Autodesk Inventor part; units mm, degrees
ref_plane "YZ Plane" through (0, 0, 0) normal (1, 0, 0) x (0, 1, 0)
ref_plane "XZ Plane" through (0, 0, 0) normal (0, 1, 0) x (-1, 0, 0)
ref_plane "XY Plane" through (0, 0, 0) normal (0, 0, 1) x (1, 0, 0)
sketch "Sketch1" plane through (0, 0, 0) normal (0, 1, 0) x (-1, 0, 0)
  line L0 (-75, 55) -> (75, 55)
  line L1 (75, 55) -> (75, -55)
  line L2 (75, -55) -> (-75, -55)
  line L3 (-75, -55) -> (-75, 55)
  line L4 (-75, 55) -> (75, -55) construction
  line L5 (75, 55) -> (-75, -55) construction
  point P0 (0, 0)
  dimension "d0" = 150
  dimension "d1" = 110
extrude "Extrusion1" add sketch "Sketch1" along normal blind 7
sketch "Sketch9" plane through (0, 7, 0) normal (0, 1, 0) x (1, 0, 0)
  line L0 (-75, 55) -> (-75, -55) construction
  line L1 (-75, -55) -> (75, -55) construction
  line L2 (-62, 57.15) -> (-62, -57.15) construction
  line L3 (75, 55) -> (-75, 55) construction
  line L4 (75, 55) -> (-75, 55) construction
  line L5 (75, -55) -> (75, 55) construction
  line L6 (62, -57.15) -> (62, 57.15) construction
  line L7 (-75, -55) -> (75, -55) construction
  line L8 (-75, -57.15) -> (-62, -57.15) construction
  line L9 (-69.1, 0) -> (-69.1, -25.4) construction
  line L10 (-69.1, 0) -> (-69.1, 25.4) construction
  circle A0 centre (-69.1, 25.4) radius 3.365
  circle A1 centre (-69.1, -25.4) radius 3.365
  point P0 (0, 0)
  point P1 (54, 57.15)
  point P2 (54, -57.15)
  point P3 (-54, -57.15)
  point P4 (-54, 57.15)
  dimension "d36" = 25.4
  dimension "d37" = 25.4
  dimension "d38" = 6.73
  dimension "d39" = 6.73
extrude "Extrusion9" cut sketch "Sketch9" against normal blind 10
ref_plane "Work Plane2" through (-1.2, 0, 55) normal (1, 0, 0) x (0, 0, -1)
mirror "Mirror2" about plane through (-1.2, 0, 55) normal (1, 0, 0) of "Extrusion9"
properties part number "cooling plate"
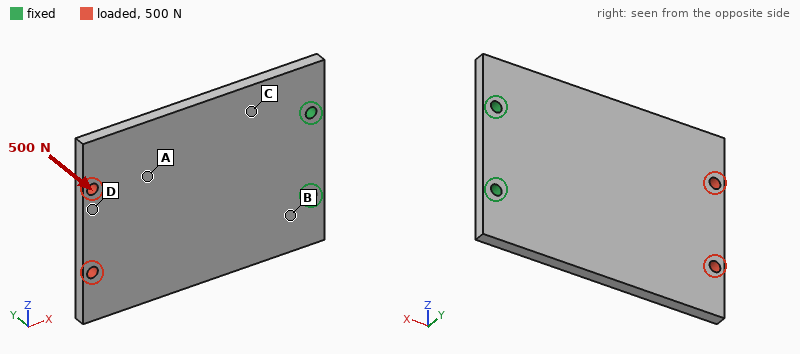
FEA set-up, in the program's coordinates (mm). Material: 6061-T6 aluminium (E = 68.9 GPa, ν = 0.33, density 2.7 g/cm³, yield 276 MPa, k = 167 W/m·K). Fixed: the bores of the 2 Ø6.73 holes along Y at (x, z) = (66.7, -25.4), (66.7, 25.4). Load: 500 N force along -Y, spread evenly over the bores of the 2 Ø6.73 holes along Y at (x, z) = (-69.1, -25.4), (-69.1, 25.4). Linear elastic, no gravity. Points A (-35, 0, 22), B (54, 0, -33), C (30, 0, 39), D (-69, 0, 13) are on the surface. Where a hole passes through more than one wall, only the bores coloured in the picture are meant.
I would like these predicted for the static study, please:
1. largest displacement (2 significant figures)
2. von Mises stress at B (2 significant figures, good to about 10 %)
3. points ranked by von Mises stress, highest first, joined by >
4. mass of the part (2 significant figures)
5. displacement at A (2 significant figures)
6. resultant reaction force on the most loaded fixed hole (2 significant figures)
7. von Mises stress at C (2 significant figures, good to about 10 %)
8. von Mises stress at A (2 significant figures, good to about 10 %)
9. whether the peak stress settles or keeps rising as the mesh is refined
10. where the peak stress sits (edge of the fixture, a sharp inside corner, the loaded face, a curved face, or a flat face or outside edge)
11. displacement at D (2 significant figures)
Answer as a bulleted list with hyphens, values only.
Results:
- 2.2 mm
- 70 MPa
- B > C > A > D
- 310 g
- 1.3 mm
- 250 N
- 53 MPa
- 20 MPa
- keeps rising
- edge of the fixture
- 2.1 mm
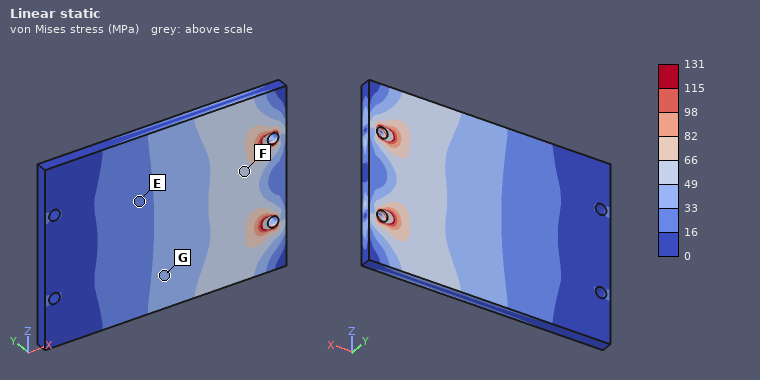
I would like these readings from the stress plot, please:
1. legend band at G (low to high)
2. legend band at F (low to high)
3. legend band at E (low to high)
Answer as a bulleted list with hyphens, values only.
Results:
- 33 to 49 MPa
- 49 to 66 MPa
- 16 to 33 MPa
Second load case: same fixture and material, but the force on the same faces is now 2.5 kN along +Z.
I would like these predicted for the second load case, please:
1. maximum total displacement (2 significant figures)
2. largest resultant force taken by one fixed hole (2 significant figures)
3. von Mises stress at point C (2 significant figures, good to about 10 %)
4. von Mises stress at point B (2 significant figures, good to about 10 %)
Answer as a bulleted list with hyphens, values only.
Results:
- 0.13 mm
- 6.2 kN
- 13 MPa
- 26 MPa
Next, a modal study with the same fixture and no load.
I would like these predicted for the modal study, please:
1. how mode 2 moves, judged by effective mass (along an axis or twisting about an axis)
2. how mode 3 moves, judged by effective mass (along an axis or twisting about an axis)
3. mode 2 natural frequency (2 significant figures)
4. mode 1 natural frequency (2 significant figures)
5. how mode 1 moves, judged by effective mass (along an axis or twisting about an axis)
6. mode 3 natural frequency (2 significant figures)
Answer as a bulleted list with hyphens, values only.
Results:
- twisting about X
- along Y
- 790 Hz
- 270 Hz
- along Y
- 1700 Hz
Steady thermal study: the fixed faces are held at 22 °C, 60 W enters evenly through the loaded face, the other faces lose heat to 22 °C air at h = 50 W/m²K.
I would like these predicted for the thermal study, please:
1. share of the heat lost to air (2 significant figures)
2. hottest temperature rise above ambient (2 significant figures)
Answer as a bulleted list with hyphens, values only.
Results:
- 56 %
- 49 K
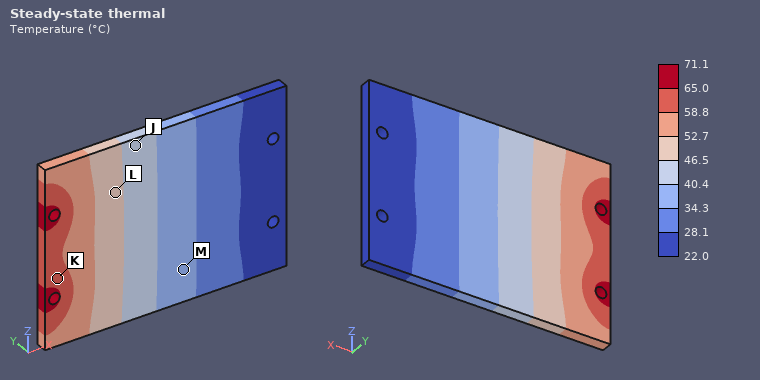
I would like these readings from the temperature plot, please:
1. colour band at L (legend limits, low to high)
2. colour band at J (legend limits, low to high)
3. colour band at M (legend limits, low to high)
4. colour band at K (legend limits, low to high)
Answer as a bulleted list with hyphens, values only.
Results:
- 46.5 to 52.7 °C
- 40.4 to 46.5 °C
- 34.3 to 40.4 °C
- 58.8 to 65.0 °C
